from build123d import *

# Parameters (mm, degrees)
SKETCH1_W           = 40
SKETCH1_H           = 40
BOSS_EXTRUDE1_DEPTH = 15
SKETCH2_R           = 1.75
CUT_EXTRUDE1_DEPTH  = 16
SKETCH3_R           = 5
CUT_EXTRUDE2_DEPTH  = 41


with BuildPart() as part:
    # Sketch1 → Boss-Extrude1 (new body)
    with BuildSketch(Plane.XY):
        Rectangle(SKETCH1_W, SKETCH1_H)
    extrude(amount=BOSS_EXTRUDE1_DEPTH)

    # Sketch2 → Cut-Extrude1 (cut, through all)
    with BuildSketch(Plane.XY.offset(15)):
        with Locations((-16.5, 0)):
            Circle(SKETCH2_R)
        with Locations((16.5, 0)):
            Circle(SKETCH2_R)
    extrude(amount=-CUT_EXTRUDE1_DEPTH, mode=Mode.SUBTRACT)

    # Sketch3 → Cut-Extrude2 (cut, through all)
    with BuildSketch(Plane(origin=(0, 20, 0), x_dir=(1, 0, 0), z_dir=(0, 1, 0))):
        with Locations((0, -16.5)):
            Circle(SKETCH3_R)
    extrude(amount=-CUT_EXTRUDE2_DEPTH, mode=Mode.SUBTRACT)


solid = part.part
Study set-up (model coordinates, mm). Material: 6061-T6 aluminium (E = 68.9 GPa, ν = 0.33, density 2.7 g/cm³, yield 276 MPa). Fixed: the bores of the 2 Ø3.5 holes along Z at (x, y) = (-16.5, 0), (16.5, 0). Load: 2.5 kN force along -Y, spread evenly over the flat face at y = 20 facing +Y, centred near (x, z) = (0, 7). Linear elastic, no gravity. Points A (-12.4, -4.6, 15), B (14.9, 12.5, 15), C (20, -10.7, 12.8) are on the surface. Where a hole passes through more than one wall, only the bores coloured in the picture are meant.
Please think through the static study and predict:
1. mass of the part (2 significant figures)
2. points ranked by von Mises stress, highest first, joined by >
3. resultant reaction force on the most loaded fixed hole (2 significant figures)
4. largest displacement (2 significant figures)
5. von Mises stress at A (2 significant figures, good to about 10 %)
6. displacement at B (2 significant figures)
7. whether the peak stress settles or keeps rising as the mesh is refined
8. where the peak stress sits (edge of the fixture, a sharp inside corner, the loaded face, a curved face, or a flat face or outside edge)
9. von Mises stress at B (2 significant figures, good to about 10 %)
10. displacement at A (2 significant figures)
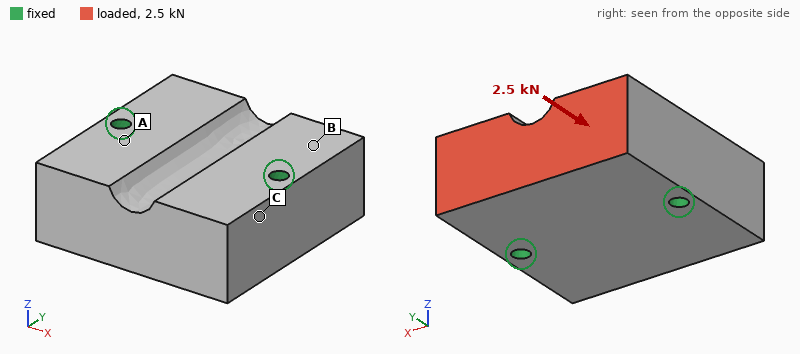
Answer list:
61 g
B > A > C
1.3 kN
2.0 µm
2.8 MPa
1.1 µm
keeps rising
edge of the fixture
4.7 MPa
0.43 µm
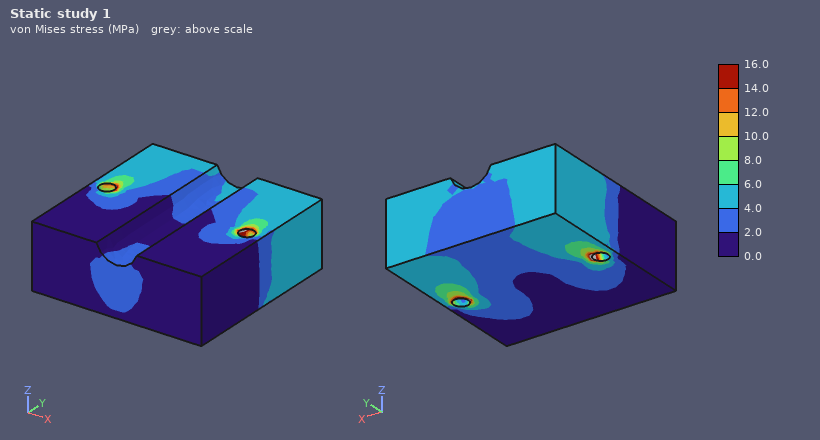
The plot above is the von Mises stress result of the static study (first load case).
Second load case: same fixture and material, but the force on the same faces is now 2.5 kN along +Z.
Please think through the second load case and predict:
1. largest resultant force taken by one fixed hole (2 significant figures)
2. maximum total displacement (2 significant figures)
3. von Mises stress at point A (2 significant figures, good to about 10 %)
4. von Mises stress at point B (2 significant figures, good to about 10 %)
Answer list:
1.3 kN
22 µm
15 MPa
16 MPa
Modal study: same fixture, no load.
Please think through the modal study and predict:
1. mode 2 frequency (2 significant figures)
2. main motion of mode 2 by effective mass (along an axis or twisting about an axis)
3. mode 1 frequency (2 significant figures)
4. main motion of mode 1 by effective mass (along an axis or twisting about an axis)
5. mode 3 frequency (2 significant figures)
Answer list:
19 kHz
along Z
16 kHz
twisting about X
27 kHz
